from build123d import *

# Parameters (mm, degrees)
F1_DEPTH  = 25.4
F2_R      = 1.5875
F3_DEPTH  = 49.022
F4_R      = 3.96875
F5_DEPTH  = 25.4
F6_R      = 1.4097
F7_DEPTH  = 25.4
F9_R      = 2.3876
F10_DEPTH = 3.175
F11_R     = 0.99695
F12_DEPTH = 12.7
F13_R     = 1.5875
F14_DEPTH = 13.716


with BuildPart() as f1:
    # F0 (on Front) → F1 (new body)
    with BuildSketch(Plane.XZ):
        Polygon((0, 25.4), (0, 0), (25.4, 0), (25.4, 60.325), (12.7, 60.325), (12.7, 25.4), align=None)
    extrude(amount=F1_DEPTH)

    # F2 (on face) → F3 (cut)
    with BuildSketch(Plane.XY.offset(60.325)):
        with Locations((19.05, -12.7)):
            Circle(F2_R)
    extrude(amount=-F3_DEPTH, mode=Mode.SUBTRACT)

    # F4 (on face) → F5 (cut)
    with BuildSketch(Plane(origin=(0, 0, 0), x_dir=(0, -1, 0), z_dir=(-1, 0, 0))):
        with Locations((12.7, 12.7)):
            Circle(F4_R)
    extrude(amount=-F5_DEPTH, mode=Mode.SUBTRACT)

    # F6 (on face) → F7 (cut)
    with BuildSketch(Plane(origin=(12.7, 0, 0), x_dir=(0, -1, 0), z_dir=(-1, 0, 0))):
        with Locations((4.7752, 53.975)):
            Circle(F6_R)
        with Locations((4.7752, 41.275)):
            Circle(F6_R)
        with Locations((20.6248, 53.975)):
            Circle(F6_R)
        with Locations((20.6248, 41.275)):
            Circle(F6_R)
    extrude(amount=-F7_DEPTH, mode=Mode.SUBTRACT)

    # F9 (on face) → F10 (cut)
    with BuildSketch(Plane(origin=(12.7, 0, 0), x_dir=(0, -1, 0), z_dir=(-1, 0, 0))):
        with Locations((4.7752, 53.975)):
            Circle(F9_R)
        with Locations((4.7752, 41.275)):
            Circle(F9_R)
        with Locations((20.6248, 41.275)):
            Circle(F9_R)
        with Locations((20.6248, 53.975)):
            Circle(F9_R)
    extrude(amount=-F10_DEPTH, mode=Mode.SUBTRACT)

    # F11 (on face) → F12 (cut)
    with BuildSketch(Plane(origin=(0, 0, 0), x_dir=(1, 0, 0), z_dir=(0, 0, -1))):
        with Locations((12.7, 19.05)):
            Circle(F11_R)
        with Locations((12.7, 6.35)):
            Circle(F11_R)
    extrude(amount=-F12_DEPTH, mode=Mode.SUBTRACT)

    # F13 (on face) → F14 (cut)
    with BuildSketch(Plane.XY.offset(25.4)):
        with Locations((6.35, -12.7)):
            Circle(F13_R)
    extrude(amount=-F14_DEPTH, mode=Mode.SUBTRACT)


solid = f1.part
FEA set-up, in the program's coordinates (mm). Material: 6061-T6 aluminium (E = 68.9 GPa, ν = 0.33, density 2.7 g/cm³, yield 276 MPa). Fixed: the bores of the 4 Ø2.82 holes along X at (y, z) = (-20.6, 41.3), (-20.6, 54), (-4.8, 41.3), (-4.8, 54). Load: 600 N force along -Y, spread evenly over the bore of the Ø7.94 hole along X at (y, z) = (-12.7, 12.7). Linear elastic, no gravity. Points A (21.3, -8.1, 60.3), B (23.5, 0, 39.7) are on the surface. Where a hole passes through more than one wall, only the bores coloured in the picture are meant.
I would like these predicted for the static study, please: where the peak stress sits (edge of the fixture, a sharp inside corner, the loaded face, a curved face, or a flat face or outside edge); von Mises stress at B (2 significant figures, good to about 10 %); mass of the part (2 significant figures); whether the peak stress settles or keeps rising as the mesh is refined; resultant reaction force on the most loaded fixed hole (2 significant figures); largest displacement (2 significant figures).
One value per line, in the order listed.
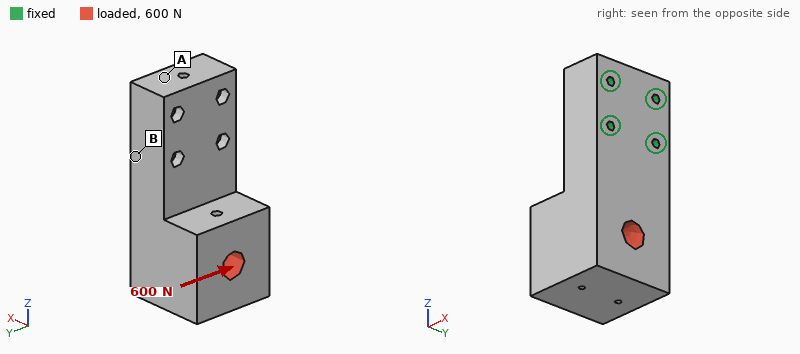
edge of the fixture
9.5 MPa
69 g
keeps rising
910 N
14 µm
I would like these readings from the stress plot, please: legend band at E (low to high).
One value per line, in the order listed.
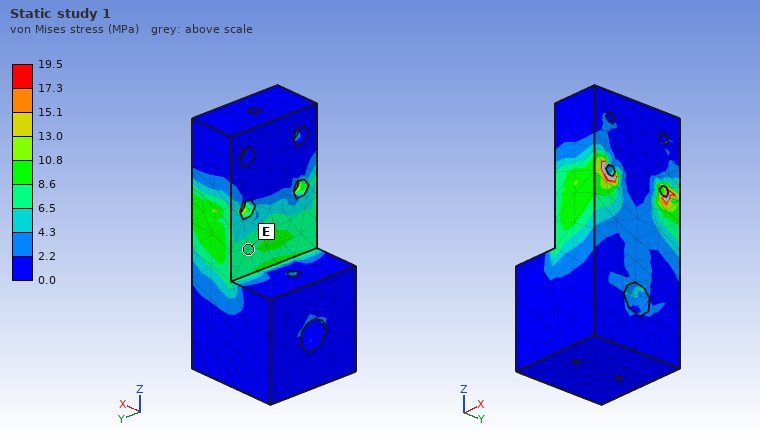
6.5 to 8.6 MPa
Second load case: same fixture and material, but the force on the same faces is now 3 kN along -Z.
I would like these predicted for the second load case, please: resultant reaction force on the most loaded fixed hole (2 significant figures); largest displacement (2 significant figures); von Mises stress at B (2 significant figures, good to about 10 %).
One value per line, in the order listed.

1.1 kN
66 µm
11 MPa
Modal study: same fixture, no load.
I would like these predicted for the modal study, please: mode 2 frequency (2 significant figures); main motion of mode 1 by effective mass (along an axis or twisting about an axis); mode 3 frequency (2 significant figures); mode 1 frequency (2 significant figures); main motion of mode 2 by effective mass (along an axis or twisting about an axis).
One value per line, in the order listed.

6300 Hz
along X
9700 Hz
3500 Hz
along Y
